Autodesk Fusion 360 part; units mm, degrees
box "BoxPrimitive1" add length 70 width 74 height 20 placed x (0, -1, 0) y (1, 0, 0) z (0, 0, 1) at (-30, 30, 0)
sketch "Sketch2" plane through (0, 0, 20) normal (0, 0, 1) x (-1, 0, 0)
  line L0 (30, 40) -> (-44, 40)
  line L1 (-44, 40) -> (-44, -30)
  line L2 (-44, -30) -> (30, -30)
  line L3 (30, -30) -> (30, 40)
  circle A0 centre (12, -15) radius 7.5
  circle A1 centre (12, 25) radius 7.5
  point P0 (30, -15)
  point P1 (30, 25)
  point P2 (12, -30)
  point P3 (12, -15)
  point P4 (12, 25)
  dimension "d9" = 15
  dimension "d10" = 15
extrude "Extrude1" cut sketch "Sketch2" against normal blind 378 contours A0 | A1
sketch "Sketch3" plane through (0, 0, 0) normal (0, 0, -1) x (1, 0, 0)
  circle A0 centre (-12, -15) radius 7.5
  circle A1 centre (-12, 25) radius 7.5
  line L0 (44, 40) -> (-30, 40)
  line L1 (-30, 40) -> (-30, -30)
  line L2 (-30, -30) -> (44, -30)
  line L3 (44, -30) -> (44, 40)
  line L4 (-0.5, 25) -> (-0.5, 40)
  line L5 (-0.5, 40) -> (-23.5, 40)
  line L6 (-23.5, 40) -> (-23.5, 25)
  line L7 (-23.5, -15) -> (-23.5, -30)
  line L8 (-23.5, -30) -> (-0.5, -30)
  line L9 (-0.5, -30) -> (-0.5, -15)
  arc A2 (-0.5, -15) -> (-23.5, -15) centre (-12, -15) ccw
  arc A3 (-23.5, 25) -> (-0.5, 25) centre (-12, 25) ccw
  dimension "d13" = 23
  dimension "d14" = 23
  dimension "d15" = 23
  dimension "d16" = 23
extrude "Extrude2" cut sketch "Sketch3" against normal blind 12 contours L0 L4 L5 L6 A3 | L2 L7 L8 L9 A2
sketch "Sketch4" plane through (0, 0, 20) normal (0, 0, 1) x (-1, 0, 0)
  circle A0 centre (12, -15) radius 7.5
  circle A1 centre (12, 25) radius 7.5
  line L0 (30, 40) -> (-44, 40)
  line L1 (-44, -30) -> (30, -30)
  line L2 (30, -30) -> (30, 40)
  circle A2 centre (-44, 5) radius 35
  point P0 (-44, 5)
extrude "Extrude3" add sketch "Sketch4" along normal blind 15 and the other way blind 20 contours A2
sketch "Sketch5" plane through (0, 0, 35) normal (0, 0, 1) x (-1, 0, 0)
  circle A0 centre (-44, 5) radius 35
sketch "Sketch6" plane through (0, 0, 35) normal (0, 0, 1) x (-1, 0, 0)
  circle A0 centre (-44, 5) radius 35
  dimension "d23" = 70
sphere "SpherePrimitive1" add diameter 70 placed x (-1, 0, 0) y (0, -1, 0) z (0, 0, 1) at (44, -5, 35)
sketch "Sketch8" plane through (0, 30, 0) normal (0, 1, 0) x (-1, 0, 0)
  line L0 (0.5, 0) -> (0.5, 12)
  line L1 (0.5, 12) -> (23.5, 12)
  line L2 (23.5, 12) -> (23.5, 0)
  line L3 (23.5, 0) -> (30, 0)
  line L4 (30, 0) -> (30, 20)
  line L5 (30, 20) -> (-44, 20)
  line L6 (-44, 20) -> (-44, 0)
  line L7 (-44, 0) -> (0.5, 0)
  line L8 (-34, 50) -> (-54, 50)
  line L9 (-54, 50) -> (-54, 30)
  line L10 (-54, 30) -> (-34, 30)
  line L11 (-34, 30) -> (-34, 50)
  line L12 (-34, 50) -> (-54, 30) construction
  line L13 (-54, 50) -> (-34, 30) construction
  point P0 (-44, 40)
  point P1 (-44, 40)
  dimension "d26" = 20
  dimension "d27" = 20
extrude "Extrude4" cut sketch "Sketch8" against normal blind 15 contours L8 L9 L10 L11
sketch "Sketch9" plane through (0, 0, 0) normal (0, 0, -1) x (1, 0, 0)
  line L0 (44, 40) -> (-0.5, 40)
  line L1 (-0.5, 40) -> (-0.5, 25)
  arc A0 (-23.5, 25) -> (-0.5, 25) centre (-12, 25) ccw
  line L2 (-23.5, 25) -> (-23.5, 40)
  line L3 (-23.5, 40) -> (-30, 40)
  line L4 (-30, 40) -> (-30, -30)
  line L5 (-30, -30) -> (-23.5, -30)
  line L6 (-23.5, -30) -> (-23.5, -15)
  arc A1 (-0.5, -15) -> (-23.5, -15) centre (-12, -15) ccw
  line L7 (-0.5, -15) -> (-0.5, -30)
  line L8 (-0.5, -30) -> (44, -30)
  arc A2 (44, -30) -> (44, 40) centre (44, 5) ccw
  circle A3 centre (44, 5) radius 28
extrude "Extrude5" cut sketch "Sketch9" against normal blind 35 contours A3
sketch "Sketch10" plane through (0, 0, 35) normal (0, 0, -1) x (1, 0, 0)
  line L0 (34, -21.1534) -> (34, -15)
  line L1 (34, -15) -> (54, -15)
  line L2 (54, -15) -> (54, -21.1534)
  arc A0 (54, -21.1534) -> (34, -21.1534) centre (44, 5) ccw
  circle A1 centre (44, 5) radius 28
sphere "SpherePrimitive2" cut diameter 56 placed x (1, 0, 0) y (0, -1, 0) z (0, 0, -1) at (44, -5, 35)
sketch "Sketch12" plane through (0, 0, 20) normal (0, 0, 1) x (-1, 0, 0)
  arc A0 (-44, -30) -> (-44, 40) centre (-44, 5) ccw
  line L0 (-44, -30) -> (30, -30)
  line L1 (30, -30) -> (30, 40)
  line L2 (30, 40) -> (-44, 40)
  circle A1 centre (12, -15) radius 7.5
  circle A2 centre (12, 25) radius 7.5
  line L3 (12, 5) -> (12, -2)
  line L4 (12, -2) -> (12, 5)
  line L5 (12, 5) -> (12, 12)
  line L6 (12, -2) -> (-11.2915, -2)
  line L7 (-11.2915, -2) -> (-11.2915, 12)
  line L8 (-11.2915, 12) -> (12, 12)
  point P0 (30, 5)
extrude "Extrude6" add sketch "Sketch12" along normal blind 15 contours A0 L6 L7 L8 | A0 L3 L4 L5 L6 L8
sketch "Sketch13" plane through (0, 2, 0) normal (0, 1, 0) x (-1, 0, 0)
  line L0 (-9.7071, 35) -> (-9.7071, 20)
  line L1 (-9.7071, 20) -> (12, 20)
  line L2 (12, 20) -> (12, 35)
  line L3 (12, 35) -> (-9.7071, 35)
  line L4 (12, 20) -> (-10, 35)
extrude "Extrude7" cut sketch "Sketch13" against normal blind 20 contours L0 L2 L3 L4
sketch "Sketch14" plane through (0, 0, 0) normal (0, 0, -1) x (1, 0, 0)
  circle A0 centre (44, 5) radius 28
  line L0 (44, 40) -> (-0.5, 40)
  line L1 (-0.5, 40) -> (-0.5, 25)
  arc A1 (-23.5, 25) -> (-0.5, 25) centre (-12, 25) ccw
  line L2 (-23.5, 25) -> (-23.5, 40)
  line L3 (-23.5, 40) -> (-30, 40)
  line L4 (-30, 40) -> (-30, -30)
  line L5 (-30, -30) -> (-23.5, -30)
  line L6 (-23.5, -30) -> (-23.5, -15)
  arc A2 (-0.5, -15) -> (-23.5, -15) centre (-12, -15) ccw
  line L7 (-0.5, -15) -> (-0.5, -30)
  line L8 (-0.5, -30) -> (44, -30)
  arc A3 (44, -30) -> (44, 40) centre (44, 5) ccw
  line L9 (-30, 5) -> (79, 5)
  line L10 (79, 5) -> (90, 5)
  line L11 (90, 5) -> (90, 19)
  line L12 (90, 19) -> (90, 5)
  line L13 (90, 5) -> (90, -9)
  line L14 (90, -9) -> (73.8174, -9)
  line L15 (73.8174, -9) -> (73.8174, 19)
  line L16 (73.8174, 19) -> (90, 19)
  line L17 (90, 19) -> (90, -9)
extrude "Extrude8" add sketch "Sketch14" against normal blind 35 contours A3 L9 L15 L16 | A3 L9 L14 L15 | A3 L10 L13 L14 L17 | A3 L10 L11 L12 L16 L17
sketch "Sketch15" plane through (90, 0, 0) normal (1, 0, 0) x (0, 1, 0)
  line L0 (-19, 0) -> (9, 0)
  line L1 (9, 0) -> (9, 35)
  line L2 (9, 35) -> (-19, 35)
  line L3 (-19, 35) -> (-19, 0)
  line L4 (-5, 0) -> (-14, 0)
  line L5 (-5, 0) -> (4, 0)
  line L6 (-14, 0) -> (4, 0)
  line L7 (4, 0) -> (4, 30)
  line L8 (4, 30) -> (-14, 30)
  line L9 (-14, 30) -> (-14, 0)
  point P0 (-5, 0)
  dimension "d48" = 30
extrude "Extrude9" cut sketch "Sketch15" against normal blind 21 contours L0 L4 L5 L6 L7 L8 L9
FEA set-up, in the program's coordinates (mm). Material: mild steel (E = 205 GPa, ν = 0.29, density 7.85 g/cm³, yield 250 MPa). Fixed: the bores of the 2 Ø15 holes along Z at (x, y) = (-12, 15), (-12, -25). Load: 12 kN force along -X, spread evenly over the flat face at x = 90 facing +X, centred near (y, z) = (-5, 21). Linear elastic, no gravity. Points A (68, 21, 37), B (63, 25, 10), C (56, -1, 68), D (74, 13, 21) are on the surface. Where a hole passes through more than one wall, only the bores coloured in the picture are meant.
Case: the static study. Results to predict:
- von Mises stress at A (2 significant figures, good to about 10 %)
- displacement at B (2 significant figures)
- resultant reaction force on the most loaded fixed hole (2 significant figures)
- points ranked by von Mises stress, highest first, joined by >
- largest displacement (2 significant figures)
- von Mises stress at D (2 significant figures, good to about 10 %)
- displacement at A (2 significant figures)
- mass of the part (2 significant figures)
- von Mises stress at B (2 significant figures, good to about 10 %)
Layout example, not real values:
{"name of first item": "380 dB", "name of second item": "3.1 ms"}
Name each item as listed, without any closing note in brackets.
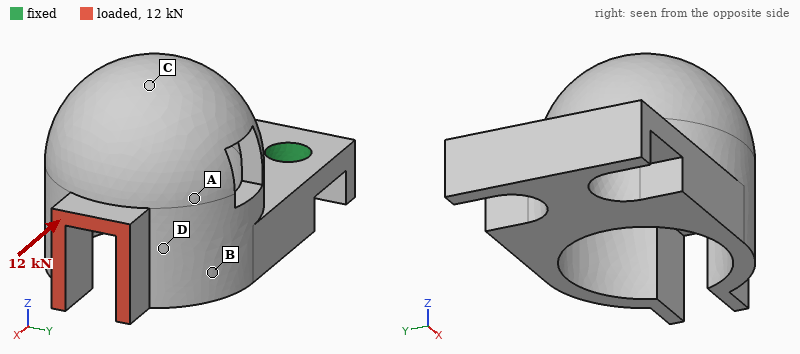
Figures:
{"von Mises stress at A": "37 MPa", "displacement at B": "32 µm", "resultant reaction force on the most loaded fixed hole": "6.2 kN", "points ranked by von Mises stress, highest first, joined by >": "D > B > A > C", "largest displacement": "93 µm", "von Mises stress at D": "100 MPa", "displacement at A": "37 µm", "mass of the part": "1.1 kg", "von Mises stress at B": "72 MPa"}
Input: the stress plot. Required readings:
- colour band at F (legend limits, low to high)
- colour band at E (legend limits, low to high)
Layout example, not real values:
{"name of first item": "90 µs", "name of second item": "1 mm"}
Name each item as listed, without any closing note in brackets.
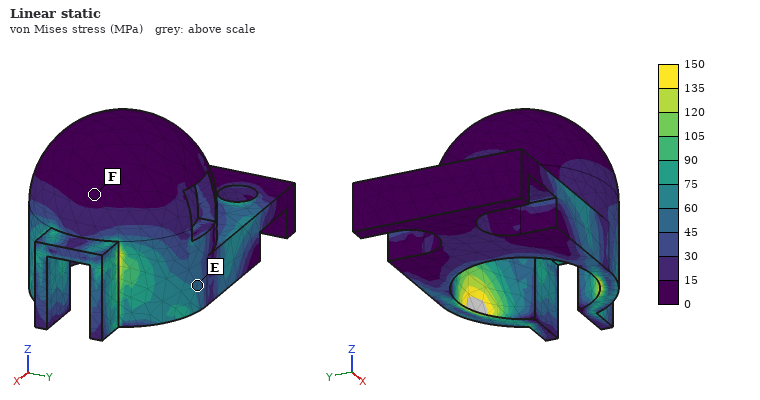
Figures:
{"colour band at F": "0 to 15 MPa", "colour band at E": "45 to 60 MPa"}
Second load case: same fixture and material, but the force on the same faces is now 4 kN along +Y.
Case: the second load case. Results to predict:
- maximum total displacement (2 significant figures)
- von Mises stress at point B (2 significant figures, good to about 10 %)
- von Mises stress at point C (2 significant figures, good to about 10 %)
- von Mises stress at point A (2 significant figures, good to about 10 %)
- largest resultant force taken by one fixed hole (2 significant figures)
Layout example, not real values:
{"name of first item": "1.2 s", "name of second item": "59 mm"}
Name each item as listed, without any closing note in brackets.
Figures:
{"maximum total displacement": "0.21 mm", "von Mises stress at point B": "46 MPa", "von Mises stress at point C": "12 MPa", "von Mises stress at point A": "25 MPa", "largest resultant force taken by one fixed hole": "8.6 kN"}
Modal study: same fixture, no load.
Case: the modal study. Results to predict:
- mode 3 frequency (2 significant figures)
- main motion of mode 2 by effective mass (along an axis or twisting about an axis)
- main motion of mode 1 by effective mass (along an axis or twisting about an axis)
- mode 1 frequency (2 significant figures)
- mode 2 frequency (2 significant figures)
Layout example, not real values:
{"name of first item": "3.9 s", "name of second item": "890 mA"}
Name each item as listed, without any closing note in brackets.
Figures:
{"mode 3 frequency": "3100 Hz", "main motion of mode 2 by effective mass": "along Y", "main motion of mode 1 by effective mass": "along Z", "mode 1 frequency": "1100 Hz", "mode 2 frequency": "2000 Hz"}
